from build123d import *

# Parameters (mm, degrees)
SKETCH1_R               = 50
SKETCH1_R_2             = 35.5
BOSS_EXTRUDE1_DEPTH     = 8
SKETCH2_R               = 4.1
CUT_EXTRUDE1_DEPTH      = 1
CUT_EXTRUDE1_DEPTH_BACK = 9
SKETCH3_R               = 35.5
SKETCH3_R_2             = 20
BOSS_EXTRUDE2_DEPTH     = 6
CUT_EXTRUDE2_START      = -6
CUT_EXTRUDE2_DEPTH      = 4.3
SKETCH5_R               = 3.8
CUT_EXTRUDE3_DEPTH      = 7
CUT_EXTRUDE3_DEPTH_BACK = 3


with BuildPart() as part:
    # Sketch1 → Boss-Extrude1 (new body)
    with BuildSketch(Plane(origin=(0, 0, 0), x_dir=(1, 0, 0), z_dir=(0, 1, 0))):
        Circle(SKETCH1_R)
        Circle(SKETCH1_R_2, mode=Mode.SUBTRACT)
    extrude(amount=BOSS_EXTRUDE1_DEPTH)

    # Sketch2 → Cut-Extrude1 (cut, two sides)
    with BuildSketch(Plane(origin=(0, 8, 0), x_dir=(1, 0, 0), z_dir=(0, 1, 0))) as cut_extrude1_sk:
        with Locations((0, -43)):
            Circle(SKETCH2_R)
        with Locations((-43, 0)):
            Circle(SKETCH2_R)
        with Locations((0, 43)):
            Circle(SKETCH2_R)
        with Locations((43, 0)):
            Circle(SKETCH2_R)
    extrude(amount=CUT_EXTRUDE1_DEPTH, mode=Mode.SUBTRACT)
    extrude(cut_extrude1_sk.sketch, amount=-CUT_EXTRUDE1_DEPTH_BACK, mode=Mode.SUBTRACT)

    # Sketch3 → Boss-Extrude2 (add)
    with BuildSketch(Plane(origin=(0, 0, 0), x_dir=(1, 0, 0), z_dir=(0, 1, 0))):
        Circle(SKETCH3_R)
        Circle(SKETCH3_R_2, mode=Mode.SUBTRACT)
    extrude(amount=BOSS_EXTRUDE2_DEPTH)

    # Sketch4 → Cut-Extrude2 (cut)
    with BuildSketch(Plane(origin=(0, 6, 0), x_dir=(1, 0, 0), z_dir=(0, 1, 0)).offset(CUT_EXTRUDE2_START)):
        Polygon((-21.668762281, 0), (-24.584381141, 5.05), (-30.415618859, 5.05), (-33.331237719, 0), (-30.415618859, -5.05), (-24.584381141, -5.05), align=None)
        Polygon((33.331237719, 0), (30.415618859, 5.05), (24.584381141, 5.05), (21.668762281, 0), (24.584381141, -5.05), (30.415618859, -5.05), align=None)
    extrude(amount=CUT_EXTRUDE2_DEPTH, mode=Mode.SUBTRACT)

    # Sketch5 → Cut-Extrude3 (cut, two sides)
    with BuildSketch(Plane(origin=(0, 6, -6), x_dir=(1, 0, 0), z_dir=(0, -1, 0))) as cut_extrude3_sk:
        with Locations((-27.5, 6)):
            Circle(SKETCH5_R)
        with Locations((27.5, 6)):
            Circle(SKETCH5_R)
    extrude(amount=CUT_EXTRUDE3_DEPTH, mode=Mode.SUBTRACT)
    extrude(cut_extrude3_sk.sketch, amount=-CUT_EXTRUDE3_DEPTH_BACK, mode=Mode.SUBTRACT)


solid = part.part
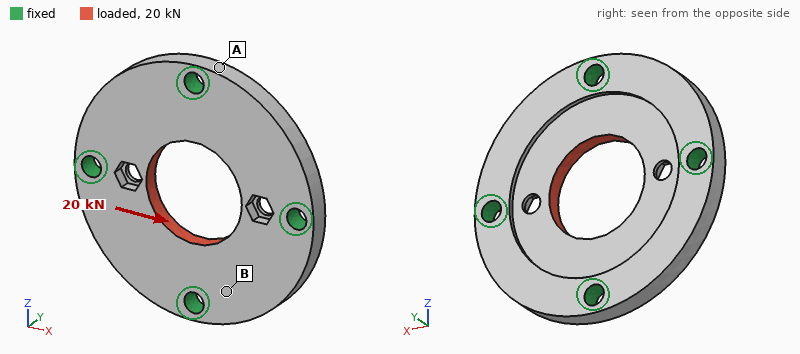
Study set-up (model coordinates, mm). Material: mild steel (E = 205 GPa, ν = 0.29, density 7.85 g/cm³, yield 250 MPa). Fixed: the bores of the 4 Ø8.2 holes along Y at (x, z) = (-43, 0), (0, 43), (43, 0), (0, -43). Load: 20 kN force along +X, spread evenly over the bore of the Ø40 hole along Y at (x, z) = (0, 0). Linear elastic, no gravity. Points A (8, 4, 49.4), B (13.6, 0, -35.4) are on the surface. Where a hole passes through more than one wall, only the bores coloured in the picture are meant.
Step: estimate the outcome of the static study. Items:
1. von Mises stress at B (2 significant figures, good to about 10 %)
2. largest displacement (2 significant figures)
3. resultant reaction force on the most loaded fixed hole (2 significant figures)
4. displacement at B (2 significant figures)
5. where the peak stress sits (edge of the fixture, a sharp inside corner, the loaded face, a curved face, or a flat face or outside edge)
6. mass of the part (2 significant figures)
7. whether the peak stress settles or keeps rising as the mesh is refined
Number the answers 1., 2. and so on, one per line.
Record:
1. 19 MPa
2. 11 µm
3. 5.2 kN
4. 2.9 µm
5. a sharp inside corner
6. 350 g
7. keeps rising
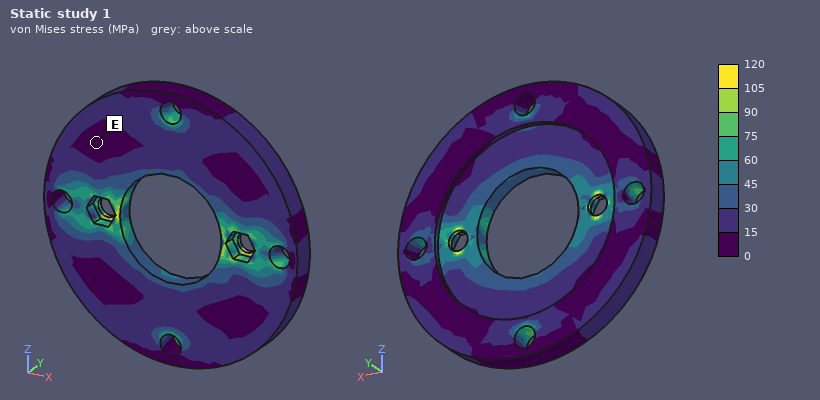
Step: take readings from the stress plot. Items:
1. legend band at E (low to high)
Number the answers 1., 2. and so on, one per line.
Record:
1. 0 to 15 MPa
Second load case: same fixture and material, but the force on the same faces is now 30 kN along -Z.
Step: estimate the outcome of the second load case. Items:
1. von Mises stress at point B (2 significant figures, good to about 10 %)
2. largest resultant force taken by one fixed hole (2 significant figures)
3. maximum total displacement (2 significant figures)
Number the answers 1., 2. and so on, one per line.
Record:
1. 32 MPa
2. 8.9 kN
3. 9.9 µm
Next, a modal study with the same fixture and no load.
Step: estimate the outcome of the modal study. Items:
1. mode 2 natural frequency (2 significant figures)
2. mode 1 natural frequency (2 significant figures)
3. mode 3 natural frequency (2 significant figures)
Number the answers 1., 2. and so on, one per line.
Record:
1. 9300 Hz
2. 9100 Hz
3. 9400 Hz
